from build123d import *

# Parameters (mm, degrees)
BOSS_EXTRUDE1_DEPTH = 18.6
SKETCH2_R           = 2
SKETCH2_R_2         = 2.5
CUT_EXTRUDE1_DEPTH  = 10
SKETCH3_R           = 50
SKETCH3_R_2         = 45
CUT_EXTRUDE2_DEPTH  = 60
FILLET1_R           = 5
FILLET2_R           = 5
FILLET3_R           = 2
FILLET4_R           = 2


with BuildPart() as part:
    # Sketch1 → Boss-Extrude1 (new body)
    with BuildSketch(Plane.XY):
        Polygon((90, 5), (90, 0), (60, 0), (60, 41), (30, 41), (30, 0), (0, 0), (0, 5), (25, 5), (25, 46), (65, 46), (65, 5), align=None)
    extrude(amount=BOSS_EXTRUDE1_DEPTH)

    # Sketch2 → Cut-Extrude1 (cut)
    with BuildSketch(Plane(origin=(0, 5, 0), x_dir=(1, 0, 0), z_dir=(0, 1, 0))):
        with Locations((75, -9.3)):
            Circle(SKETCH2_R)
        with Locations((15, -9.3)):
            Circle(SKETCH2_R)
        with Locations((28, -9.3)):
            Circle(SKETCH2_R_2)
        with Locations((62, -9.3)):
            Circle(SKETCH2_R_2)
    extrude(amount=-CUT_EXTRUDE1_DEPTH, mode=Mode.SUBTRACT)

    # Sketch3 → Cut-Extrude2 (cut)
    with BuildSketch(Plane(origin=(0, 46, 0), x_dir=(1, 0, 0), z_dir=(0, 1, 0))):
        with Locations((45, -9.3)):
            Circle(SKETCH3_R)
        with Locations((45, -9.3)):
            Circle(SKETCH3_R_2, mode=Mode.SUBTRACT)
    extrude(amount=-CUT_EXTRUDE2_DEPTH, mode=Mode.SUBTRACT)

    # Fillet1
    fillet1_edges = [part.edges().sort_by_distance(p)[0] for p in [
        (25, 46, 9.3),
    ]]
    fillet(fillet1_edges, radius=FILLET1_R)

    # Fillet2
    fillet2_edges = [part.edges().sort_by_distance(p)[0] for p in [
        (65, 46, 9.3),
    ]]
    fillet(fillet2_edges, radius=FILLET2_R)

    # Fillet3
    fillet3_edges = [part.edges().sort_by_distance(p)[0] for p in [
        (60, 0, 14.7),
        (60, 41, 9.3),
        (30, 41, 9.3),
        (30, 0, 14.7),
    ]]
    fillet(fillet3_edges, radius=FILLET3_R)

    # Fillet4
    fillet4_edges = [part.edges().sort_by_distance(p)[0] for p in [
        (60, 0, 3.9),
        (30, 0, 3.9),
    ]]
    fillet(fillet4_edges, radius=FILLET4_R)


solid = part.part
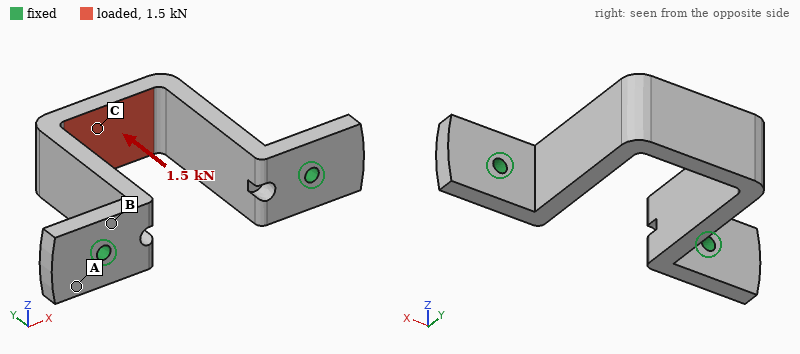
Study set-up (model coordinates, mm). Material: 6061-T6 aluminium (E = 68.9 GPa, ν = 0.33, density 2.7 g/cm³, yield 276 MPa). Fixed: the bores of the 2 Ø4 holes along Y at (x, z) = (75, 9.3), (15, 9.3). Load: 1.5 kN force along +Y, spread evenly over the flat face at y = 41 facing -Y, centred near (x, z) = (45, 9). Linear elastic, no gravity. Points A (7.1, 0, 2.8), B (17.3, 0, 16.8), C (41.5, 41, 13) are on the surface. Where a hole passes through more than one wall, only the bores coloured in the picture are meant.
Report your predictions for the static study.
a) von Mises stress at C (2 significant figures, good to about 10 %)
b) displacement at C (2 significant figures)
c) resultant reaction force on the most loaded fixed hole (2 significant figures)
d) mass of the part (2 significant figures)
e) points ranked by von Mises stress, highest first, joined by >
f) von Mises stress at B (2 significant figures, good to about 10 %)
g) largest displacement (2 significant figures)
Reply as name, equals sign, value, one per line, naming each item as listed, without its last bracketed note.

von Mises stress at C = 42 MPa
displacement at C = 53 µm
resultant reaction force on the most loaded fixed hole = 770 N
mass of the part = 42 g
points ranked by von Mises stress, highest first, joined by > = C > B > A
von Mises stress at B = 24 MPa
largest displacement = 58 µm
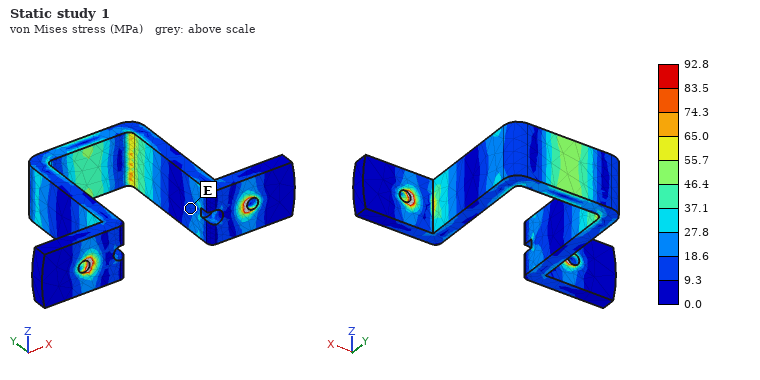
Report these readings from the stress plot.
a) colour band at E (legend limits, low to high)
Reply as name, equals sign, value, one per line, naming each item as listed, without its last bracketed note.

colour band at E = 9.3 to 18.6 MPa
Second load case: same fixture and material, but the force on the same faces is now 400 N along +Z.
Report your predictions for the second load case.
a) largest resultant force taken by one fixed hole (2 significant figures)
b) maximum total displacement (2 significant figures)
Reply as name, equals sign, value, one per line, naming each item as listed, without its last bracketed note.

largest resultant force taken by one fixed hole = 200 N
maximum total displacement = 0.23 mm
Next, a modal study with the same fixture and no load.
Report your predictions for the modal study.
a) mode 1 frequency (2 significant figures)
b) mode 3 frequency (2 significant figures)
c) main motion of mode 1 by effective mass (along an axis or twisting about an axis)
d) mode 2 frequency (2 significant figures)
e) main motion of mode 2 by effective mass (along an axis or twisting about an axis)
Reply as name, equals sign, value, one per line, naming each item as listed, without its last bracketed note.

mode 1 frequency = 1700 Hz
mode 3 frequency = 3600 Hz
main motion of mode 1 by effective mass = along Z
mode 2 frequency = 2100 Hz
main motion of mode 2 by effective mass = along X
